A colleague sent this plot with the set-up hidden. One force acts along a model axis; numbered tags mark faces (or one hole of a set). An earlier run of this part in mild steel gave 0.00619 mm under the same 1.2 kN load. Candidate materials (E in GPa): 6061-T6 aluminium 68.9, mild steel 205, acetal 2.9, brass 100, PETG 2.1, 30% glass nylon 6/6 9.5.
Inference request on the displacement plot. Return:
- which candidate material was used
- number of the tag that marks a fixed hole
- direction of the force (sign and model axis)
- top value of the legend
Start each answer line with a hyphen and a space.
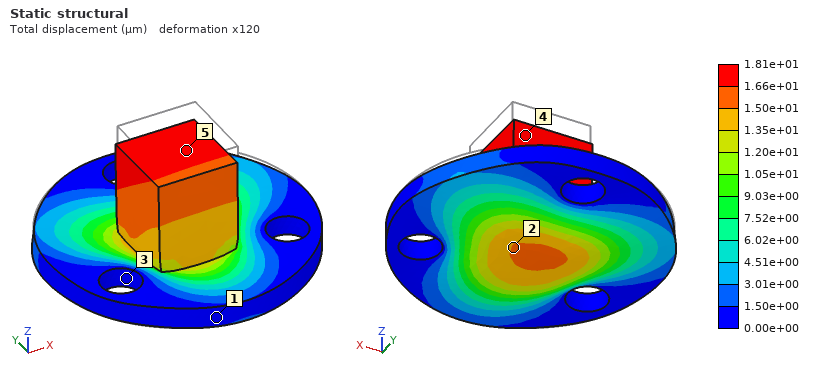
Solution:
- 6061-T6 aluminium
- 3
- -Z
- 1.81e+01 µm
